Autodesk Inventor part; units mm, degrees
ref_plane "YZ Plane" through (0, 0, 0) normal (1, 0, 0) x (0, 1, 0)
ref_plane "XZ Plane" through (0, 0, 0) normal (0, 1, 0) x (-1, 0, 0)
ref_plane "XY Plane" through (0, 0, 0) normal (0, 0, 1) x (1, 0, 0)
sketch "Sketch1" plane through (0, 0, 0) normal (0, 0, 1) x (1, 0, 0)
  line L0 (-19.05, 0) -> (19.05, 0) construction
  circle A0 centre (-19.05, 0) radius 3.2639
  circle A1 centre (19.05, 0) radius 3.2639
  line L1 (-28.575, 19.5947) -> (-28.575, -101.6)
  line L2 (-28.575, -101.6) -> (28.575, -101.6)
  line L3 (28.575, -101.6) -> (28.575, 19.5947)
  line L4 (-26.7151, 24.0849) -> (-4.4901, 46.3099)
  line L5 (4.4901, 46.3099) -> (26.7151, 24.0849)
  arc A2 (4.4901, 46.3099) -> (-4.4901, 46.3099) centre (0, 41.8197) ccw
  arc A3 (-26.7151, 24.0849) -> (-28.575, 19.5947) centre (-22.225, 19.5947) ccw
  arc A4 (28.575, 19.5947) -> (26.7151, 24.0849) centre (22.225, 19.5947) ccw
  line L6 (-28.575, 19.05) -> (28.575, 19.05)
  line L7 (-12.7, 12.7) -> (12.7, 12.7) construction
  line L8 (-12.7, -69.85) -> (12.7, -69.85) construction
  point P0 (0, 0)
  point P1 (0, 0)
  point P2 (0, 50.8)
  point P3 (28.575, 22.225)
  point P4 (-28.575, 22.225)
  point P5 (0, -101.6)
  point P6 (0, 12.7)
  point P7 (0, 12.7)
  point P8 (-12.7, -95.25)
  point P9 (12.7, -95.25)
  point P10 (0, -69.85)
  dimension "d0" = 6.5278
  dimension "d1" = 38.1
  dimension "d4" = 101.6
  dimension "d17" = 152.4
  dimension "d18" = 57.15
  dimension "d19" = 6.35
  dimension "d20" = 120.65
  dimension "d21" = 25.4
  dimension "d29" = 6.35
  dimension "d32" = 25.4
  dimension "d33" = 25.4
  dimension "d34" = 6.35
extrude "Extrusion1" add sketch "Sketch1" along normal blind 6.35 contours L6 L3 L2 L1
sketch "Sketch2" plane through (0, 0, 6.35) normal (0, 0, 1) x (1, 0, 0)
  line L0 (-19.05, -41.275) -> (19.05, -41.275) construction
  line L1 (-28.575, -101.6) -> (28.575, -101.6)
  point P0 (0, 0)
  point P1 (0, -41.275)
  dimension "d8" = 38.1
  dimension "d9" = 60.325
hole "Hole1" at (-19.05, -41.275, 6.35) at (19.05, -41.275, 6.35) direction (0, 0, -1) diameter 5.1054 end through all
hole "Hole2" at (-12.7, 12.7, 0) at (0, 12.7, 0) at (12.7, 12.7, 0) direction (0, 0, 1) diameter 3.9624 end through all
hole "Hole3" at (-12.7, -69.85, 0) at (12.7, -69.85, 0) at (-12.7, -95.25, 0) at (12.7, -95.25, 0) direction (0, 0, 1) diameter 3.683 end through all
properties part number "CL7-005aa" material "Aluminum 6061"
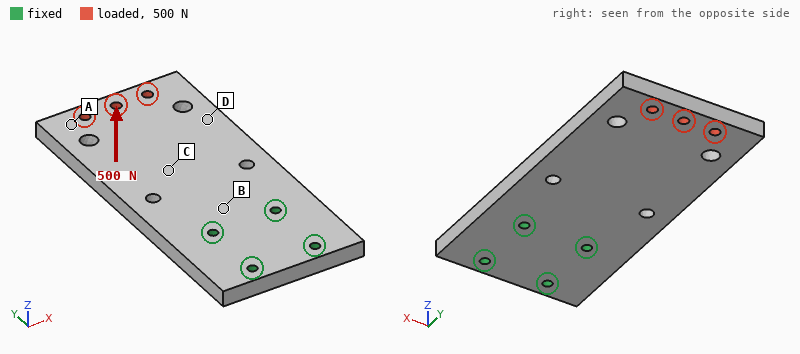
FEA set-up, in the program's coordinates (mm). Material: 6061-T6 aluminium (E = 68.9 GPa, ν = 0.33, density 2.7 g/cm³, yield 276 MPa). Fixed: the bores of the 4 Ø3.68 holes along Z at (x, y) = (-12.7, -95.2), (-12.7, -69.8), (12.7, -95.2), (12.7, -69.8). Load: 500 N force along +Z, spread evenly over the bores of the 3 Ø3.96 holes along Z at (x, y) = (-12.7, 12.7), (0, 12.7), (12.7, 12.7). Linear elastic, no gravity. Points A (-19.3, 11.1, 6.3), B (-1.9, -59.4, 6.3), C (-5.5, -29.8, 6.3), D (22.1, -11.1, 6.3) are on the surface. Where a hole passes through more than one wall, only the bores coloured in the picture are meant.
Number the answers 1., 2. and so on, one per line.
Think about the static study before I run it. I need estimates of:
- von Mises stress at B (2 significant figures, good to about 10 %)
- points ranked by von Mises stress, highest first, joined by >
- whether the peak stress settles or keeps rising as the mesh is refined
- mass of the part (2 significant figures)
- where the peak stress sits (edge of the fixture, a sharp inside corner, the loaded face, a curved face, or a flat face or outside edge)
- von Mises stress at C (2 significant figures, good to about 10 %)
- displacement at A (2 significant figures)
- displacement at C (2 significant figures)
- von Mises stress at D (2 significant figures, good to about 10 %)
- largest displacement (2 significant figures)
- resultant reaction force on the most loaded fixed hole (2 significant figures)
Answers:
1. 87 MPa
2. B > C > D > A
3. keeps rising
4. 120 g
5. edge of the fixture
6. 55 MPa
7. 1.1 mm
8. 0.37 mm
9. 30 MPa
10. 1.3 mm
11. 580 N
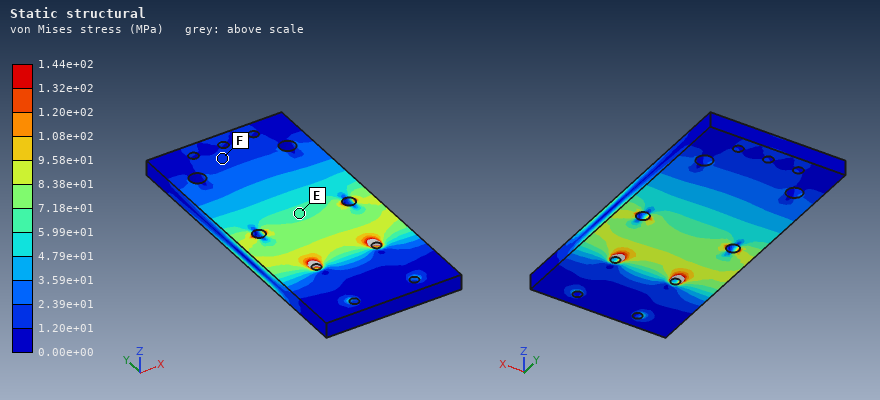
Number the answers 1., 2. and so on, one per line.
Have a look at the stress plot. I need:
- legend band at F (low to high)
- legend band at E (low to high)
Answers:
1. 1.20e+01 to 2.39e+01 MPa
2. 5.99e+01 to 7.18e+01 MPa
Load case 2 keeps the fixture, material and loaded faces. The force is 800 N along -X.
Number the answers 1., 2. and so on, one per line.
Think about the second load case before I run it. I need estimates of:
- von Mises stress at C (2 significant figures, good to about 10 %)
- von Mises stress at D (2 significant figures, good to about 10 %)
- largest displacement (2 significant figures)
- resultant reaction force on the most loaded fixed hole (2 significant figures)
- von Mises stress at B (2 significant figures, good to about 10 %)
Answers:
1. 6.0 MPa
2. 4.2 MPa
3. 49 µm
4. 1.6 kN
5. 8.5 MPa
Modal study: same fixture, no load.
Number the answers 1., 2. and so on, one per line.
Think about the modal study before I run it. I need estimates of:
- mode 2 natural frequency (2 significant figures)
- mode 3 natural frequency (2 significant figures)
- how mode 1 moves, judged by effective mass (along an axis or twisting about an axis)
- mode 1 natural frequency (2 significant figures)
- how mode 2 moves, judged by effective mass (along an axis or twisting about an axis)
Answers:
1. 2100 Hz
2. 3900 Hz
3. along Z
4. 650 Hz
5. twisting about Y
